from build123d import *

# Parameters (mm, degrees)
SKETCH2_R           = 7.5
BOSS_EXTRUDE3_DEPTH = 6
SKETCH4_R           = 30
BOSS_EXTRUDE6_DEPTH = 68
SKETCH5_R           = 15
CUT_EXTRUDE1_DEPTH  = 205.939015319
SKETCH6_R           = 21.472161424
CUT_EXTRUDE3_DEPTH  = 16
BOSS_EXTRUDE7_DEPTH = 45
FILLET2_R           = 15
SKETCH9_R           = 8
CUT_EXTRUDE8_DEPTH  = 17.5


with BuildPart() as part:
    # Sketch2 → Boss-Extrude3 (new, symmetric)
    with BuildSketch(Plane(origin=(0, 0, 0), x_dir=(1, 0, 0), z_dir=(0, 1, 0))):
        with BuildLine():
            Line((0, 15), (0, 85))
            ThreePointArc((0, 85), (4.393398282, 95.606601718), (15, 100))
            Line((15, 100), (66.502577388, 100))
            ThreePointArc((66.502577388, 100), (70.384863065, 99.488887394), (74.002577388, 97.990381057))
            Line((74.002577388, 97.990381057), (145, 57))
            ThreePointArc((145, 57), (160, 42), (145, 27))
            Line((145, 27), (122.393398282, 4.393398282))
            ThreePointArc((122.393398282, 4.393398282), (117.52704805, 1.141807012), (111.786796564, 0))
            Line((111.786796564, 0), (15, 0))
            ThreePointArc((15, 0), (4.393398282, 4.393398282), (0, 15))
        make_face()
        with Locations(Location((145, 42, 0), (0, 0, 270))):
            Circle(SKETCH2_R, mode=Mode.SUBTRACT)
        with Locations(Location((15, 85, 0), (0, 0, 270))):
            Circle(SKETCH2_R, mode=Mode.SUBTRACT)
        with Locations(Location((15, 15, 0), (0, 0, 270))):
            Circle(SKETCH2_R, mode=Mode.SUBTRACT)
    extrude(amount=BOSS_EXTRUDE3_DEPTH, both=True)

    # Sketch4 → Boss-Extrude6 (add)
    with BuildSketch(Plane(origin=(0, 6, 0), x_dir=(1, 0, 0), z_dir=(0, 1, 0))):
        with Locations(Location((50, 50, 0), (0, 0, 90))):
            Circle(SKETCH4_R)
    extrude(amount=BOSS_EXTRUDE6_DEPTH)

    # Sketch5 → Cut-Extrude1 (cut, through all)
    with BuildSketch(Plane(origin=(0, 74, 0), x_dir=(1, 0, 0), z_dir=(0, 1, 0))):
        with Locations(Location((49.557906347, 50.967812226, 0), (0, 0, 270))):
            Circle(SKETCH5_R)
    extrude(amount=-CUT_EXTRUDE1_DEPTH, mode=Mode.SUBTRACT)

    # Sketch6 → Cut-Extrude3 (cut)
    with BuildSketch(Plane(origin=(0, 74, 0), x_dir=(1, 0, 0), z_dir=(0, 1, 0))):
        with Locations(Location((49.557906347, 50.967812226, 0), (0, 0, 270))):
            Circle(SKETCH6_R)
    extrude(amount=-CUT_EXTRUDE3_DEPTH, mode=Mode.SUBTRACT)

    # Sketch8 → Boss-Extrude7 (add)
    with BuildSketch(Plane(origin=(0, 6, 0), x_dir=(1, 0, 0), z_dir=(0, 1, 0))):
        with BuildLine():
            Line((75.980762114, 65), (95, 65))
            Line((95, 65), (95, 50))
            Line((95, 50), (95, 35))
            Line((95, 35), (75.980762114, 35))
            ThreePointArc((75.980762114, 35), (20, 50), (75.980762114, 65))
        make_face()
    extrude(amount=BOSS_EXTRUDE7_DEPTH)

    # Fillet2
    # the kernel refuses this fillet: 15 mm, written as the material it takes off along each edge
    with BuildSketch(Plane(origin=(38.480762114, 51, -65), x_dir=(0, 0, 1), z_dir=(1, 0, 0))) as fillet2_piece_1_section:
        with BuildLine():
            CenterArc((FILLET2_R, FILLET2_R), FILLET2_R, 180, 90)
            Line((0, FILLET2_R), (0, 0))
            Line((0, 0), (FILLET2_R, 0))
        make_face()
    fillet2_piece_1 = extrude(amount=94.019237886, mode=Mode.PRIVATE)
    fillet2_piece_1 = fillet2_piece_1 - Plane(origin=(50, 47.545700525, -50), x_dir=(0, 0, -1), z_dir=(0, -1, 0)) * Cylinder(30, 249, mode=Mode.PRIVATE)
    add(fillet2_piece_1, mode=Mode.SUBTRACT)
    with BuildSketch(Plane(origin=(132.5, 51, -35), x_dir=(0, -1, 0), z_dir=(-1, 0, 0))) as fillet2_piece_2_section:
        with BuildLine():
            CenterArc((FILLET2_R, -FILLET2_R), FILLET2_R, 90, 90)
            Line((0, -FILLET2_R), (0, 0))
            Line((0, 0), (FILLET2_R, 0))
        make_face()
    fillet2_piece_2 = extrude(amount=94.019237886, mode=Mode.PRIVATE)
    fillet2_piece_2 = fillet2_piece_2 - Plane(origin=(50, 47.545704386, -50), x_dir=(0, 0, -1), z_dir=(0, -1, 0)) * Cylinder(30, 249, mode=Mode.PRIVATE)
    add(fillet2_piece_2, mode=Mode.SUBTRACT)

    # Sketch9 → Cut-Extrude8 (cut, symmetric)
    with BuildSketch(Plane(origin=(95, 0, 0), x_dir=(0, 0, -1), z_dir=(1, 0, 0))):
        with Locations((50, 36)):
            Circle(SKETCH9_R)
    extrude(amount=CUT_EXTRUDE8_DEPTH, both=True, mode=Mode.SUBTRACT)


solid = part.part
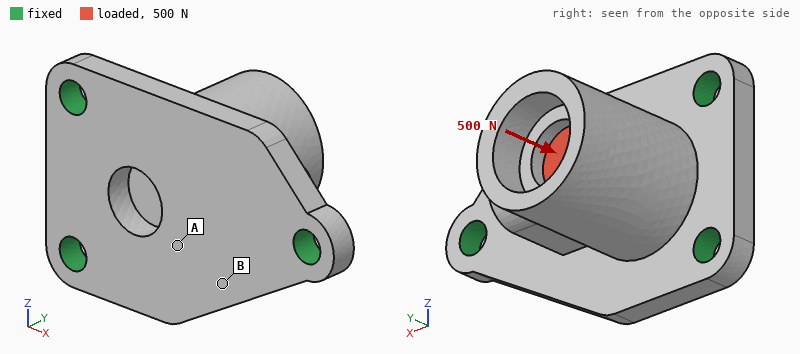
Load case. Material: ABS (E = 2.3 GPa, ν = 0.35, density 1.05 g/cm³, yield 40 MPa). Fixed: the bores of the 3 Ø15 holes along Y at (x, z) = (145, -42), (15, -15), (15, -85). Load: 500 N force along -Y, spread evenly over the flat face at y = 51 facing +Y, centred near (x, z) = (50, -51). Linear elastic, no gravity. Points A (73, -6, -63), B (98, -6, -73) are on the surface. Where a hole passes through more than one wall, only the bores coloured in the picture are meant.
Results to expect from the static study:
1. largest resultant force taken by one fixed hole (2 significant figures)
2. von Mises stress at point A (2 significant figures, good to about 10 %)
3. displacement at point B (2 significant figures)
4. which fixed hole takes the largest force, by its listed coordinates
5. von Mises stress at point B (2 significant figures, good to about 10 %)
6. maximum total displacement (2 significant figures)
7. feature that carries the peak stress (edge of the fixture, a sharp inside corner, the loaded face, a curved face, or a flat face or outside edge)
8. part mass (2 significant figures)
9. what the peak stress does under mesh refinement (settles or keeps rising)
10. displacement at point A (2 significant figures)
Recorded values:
220 N
0.41 MPa
76 µm
(15, -85)
1.0 MPa
92 µm
edge of the fixture
340 g
keeps rising
67 µm
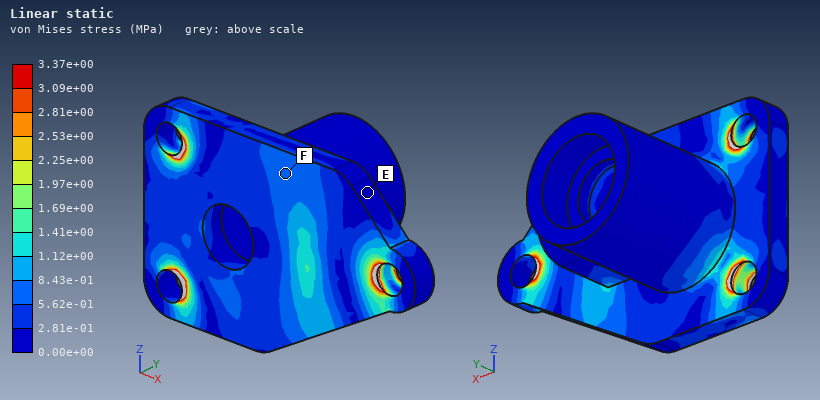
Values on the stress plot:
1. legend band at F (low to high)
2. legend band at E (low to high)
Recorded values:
5.62e-01 to 8.43e-01 MPa
0.00e+00 to 2.81e-01 MPa
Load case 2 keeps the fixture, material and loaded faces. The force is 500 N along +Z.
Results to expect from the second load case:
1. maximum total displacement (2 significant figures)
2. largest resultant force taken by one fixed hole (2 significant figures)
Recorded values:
0.20 mm
490 N
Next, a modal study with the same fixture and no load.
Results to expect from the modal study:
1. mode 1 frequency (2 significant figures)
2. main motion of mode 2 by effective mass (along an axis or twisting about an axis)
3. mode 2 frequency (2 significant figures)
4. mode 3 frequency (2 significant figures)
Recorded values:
650 Hz
along Z
820 Hz
1500 Hz
